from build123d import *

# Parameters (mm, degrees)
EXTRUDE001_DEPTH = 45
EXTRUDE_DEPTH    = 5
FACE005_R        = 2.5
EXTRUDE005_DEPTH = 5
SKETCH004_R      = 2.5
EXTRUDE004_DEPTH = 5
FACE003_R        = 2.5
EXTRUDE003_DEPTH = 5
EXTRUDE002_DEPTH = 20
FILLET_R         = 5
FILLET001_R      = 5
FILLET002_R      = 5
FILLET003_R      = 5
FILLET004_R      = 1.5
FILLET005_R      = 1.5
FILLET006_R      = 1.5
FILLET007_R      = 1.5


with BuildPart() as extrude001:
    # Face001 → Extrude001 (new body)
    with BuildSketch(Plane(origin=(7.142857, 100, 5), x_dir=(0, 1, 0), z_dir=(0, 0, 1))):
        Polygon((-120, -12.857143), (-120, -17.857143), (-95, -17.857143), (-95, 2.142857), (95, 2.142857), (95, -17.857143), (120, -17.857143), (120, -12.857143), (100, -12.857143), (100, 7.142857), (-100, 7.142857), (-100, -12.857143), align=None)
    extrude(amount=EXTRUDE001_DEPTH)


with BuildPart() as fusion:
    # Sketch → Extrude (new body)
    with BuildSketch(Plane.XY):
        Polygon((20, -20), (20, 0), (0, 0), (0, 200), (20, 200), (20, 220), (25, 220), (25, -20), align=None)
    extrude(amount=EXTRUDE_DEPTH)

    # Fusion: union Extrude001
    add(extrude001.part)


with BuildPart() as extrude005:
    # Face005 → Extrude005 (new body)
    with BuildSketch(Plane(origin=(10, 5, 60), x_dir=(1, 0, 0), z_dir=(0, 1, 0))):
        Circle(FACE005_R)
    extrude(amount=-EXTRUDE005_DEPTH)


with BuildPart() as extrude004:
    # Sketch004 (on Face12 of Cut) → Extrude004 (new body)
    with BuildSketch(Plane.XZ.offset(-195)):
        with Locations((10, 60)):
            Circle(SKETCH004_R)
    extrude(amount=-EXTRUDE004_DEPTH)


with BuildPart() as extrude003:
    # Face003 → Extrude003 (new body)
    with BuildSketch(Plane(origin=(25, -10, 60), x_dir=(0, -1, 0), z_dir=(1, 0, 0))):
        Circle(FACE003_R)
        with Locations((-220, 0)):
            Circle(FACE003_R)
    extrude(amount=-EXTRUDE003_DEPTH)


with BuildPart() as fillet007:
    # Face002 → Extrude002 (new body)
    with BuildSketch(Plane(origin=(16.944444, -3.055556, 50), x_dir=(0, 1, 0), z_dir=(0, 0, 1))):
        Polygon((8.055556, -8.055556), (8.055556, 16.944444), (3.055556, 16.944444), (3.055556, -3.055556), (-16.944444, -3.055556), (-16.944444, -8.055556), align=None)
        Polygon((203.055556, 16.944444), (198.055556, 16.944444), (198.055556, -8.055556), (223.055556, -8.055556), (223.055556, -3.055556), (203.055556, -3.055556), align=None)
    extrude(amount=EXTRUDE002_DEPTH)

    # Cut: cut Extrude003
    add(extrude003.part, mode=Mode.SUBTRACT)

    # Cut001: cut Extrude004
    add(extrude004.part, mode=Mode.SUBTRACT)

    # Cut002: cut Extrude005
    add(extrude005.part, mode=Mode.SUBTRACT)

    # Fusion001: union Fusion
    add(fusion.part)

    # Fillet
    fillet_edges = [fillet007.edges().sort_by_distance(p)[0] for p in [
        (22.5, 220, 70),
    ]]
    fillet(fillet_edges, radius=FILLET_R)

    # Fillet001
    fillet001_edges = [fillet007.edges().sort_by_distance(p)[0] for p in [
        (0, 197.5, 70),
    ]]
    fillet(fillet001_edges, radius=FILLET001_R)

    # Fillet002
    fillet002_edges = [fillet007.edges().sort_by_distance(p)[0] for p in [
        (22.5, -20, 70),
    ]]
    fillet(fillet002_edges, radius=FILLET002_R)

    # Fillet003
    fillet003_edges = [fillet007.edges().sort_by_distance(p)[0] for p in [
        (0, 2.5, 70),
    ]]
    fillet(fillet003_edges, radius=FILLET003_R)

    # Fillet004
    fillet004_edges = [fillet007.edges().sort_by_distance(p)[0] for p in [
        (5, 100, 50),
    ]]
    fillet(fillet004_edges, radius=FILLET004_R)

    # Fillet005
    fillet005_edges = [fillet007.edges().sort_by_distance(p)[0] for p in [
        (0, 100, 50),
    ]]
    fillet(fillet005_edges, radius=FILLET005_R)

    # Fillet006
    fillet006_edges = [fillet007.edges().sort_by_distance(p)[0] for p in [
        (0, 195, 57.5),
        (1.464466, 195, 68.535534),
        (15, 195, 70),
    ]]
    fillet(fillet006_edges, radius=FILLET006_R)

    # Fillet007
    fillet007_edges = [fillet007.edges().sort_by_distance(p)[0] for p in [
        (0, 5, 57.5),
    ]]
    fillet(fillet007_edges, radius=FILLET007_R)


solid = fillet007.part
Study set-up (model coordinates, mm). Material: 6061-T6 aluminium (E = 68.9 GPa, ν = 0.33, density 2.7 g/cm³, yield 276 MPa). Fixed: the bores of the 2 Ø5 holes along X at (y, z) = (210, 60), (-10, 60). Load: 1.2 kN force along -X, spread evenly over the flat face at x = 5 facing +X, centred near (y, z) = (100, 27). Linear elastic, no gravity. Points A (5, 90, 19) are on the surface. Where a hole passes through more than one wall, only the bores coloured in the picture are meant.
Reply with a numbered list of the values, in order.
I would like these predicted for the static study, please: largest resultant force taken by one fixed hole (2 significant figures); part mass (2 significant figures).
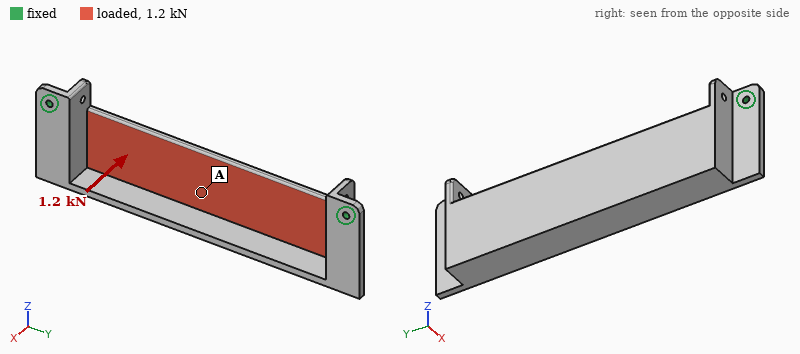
1. 790 N
2. 260 g
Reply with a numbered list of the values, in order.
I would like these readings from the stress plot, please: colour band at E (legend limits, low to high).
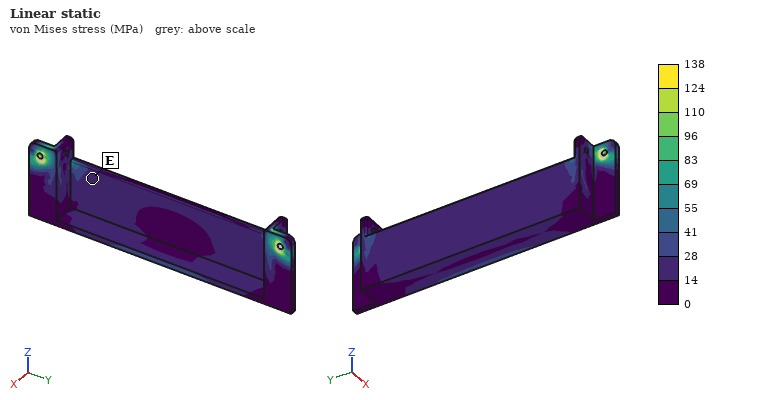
1. 14 to 28 MPa
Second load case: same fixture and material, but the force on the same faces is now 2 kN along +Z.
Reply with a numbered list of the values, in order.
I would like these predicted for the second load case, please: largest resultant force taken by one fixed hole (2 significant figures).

1. 1.0 kN
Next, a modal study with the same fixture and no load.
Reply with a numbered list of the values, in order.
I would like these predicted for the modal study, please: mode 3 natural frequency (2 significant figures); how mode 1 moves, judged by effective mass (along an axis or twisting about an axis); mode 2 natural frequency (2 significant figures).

1. 1200 Hz
2. along X
3. 1000 Hz
